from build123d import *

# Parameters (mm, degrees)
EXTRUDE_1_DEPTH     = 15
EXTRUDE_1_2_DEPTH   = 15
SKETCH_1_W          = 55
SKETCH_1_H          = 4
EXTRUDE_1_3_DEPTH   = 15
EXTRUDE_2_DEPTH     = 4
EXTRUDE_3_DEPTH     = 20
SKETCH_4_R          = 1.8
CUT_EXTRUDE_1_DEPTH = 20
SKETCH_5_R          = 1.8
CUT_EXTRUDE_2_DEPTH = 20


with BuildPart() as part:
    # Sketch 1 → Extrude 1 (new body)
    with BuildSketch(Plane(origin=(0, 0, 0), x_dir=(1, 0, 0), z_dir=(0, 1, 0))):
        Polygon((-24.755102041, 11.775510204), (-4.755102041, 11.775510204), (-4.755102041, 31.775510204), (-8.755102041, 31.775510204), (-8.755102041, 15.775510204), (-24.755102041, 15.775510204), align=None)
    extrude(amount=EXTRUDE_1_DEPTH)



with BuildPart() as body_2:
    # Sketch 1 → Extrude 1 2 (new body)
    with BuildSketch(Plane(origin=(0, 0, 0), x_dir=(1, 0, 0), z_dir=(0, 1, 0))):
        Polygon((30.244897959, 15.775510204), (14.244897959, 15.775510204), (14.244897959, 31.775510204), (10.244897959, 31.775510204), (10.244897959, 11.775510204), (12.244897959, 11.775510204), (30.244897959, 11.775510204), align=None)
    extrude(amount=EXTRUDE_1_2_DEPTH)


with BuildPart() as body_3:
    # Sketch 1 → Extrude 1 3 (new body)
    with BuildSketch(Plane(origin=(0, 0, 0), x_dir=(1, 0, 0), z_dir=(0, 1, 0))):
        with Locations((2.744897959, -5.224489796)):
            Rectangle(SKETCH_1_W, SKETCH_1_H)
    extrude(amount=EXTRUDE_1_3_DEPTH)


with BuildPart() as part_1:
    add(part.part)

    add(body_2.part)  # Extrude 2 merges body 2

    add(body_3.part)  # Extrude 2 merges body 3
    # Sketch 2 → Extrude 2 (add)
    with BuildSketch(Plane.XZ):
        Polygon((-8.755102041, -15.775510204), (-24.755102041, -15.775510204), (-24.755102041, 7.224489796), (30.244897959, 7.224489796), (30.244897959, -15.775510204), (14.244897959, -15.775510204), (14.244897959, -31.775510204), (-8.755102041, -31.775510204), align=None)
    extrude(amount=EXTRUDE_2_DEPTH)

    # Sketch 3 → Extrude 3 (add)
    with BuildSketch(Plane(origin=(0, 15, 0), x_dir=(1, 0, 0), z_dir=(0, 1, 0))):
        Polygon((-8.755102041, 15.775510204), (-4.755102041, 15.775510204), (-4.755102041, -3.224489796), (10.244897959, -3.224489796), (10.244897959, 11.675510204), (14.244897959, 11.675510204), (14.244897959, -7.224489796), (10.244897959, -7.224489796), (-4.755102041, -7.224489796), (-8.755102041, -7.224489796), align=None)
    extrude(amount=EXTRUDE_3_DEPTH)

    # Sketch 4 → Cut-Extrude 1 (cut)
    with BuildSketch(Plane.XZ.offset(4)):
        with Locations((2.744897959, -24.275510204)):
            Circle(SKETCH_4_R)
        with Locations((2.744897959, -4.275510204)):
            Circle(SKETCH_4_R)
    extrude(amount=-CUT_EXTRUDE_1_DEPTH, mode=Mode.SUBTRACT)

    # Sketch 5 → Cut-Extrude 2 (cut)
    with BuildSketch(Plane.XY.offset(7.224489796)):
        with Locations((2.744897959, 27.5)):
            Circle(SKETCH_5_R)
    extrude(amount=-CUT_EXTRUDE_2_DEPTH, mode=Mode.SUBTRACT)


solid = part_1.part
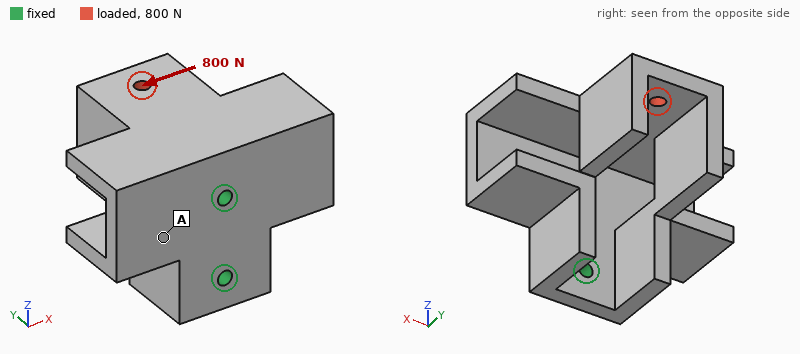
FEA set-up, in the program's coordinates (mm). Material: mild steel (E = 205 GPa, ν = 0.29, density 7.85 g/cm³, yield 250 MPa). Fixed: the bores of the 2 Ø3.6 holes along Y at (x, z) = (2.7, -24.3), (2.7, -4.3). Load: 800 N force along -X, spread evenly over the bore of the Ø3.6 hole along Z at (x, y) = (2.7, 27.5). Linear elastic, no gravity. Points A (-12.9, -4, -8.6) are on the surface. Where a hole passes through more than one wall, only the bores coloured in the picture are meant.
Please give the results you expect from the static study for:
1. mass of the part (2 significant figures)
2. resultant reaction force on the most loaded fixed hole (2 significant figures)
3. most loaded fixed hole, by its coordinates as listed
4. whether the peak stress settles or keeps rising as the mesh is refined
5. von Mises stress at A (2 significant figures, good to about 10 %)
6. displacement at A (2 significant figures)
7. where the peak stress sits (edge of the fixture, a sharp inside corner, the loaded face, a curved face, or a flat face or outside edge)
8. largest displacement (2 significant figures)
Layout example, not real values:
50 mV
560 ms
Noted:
150 g
1.1 kN
(2.7, -4.3)
keeps rising
34 MPa
0.034 mm
edge of the fixture
0.14 mm
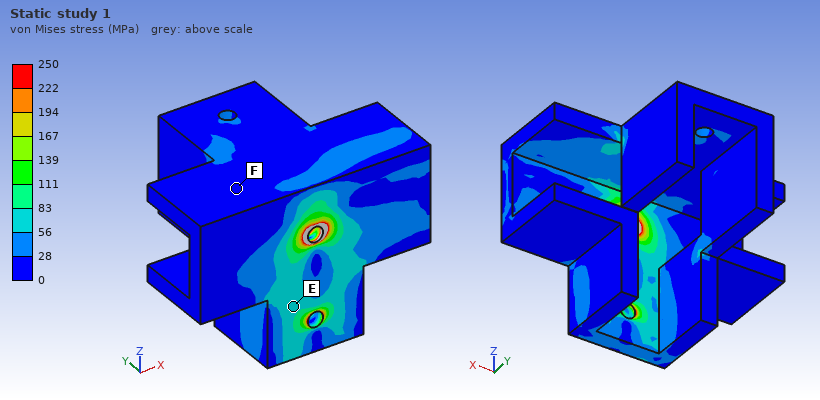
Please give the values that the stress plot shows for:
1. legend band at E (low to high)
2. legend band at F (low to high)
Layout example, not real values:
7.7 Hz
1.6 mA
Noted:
56 to 83 MPa
0 to 28 MPa
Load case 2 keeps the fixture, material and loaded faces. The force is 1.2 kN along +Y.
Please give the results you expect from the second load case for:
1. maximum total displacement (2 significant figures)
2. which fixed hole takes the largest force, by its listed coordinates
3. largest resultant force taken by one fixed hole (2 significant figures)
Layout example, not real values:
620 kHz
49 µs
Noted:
25 µm
(2.7, -4.3)
1.5 kN
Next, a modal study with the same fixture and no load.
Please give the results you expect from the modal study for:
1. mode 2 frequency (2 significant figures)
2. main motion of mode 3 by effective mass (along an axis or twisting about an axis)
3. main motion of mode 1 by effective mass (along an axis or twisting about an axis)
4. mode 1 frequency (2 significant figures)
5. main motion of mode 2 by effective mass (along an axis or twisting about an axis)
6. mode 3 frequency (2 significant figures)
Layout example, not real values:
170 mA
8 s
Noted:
3100 Hz
along Y
along X
1900 Hz
along Z
5100 Hz
